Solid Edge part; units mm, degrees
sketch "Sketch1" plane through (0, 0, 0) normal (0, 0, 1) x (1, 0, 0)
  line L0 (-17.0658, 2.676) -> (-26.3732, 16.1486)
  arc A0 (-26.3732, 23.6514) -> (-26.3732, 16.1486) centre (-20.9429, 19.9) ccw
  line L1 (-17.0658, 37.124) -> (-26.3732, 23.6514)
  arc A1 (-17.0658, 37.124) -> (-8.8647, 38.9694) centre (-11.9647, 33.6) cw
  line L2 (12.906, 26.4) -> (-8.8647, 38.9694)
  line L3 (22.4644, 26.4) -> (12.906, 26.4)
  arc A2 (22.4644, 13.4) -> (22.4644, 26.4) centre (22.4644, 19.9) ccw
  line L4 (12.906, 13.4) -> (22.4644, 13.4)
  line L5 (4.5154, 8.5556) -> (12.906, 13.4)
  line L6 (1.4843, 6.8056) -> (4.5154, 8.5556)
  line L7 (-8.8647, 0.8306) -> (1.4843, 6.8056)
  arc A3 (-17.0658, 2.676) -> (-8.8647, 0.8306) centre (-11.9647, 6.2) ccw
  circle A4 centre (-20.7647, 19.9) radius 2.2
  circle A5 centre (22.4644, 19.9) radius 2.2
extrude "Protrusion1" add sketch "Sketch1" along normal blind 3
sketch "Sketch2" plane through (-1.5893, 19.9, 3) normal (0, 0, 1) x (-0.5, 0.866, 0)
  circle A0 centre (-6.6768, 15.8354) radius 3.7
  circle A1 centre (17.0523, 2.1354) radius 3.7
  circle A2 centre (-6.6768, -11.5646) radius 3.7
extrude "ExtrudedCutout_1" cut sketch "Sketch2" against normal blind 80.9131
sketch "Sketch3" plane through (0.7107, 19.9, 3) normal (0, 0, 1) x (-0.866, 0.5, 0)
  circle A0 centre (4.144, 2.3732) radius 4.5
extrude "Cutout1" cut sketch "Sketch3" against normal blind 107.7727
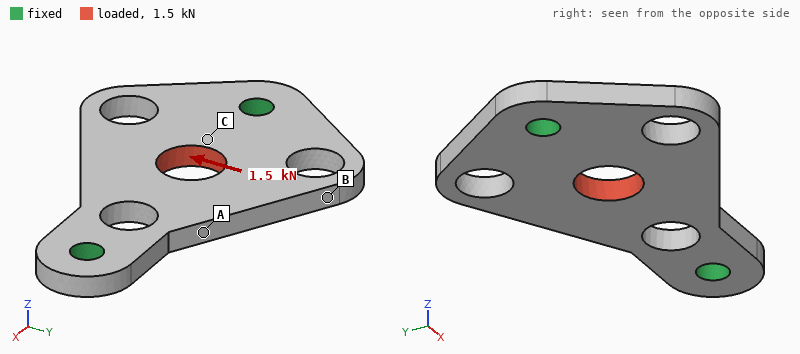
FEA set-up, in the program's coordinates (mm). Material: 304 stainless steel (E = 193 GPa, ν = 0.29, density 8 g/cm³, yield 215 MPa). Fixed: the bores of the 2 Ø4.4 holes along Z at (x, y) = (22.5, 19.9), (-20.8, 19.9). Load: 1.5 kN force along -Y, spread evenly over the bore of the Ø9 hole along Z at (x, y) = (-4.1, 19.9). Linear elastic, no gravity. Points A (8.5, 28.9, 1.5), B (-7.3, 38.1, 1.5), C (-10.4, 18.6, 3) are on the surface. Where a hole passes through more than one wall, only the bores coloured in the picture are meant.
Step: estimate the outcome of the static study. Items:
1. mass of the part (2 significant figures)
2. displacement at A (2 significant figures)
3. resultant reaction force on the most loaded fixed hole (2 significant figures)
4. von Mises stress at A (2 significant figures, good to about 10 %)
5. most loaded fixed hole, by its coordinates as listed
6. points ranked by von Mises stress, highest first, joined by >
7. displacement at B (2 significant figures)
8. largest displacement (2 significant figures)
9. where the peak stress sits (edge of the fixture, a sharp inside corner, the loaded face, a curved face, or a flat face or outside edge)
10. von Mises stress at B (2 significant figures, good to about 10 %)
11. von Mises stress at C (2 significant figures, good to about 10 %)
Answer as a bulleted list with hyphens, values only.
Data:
- 25 g
- 7.1 µm
- 960 N
- 64 MPa
- (-20.8, 19.9)
- A > C > B
- 6.7 µm
- 8.1 µm
- edge of the fixture
- 18 MPa
- 35 MPa
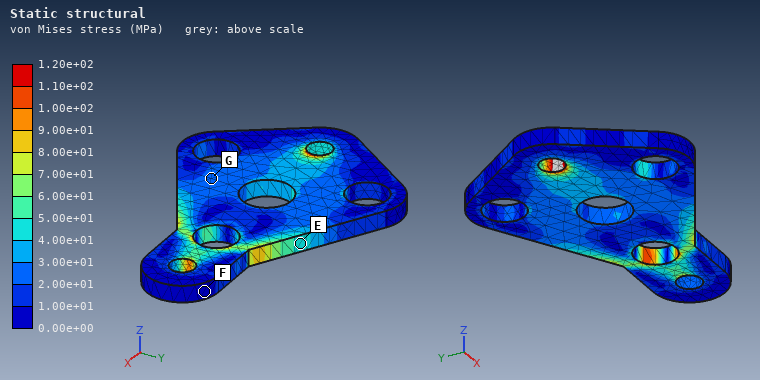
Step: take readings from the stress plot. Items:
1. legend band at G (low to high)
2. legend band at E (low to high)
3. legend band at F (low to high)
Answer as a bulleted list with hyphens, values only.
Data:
- 2.00e+01 to 3.00e+01 MPa
- 4.00e+01 to 5.00e+01 MPa
- 0.00e+00 to 1.00e+01 MPa
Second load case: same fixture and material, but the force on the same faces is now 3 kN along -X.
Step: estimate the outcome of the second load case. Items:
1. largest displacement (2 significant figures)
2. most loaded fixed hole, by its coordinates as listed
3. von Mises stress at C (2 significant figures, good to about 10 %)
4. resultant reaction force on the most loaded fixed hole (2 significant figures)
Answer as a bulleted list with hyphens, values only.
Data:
- 5.4 µm
- (-20.8, 19.9)
- 49 MPa
- 2.0 kN
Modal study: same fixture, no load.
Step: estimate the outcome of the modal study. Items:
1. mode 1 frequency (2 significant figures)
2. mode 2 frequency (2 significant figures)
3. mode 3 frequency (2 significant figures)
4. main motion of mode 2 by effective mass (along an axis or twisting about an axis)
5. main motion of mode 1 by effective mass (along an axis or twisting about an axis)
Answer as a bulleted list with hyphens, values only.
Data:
- 5900 Hz
- 6500 Hz
- 12 kHz
- along Z
- twisting about X
